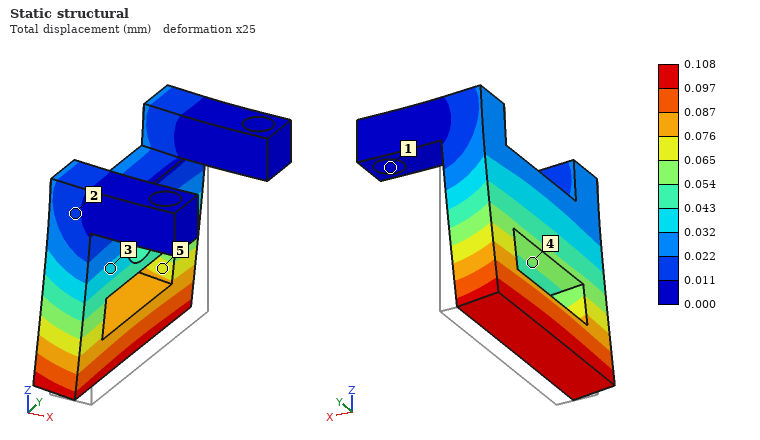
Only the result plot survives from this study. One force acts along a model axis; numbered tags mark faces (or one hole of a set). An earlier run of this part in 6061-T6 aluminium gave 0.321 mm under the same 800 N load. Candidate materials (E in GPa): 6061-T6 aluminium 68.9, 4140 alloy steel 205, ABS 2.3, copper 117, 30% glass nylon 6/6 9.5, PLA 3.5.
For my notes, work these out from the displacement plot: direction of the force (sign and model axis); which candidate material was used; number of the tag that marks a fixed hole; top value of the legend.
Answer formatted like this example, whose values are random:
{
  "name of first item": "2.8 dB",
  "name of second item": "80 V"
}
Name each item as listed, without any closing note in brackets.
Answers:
{
  "direction of the force": "-X",
  "which candidate material was used": "4140 alloy steel",
  "number of the tag that marks a fixed hole": "1",
  "top value of the legend": "0.108 mm"
}
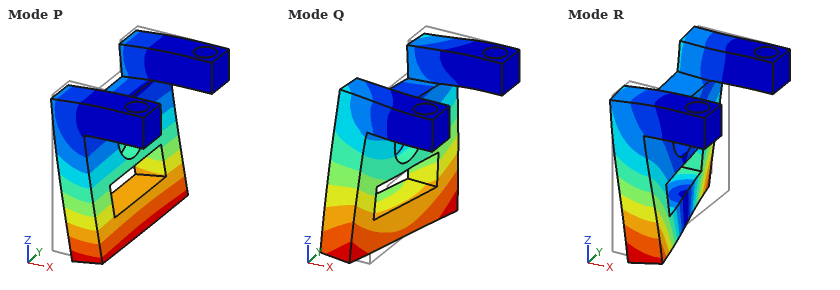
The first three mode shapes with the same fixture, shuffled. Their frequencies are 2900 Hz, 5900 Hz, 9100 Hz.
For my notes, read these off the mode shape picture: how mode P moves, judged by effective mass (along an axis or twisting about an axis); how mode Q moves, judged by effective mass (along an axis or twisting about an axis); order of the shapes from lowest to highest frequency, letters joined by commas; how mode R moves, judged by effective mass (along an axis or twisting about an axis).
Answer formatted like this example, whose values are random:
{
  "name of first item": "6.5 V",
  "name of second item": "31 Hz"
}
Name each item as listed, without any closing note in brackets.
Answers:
{
  "how mode P moves, judged by effective mass": "along X",
  "how mode Q moves, judged by effective mass": "along Y",
  "order of the shapes from lowest to highest frequency, letters joined by commas": "P, Q, R",
  "how mode R moves, judged by effective mass": "along Y"
}
